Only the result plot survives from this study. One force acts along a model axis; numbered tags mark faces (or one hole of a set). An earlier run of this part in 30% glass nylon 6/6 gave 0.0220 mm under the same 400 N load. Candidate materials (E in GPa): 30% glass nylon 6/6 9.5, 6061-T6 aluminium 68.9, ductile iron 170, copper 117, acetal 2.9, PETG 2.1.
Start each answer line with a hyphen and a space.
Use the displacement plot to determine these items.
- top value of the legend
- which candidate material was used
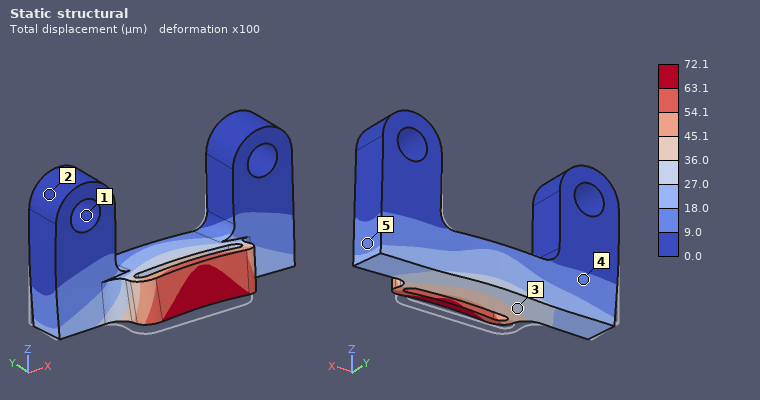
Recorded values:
- 72.1 µm
- acetal
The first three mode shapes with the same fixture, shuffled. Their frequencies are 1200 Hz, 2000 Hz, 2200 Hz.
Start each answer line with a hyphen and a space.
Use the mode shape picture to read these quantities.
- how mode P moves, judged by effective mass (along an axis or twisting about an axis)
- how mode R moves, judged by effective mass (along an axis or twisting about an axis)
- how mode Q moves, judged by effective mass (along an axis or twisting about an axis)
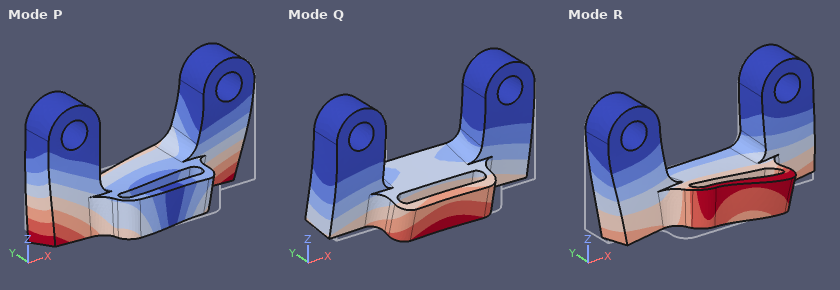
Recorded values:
- along X
- along X
- along Y
